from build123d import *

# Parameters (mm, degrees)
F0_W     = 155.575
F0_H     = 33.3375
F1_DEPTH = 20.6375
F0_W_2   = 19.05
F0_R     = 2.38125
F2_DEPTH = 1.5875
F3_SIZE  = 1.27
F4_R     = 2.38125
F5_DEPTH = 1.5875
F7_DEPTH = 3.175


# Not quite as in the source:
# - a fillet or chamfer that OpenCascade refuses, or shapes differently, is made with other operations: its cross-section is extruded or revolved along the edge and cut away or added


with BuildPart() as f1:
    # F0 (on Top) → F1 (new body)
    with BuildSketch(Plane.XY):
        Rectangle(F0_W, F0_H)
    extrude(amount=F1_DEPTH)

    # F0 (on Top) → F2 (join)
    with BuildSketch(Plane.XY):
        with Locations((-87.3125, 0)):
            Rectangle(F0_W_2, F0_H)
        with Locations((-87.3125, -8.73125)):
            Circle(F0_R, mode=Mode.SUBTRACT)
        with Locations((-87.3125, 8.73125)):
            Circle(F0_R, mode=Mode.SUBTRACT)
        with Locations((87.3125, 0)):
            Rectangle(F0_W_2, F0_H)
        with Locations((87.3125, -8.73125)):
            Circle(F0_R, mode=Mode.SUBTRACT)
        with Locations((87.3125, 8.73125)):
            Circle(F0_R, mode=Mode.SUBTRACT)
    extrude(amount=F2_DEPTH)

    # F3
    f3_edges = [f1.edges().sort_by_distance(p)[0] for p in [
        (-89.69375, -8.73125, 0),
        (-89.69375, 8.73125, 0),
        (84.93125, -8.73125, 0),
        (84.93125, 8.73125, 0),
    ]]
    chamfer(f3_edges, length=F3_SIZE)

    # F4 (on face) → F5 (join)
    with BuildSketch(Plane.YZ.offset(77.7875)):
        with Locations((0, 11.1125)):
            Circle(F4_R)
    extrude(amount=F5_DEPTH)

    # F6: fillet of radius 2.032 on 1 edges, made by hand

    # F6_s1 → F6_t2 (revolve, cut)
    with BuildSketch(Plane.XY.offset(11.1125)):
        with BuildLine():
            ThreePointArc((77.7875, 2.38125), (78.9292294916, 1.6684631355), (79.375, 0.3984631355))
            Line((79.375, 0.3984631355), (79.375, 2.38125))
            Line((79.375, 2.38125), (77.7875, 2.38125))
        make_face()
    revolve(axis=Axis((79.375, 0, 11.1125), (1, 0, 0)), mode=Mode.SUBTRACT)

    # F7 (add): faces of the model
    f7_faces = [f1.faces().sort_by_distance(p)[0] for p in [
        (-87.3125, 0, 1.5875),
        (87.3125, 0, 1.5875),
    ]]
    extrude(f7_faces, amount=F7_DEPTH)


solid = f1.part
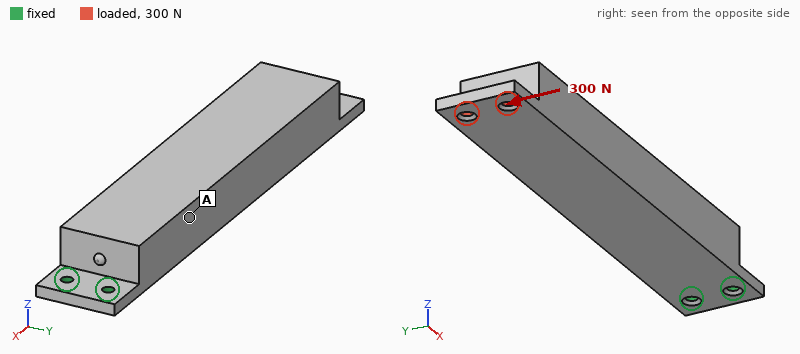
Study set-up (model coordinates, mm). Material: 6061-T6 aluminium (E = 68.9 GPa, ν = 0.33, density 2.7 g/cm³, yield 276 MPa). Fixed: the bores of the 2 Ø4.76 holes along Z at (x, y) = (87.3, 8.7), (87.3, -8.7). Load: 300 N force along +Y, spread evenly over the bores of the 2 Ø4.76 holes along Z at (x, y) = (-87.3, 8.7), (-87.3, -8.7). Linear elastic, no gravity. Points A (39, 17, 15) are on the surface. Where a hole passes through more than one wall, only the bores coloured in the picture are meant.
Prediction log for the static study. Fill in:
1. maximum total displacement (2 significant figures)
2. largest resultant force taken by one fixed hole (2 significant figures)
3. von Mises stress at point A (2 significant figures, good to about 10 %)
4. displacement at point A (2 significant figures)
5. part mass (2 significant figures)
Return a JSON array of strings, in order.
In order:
["0.30 mm", "2.6 kN", "9.6 MPa", "0.054 mm", "300 g"]
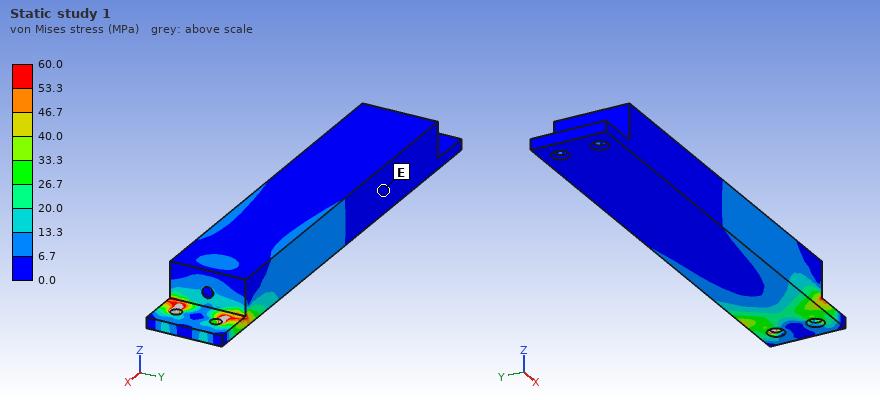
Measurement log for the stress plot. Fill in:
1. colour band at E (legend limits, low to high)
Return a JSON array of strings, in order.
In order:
["0.0 to 6.7 MPa"]
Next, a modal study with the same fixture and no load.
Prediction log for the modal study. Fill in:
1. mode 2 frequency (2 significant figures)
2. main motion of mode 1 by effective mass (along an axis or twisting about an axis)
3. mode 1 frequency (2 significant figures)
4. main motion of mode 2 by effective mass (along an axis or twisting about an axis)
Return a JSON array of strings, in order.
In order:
["570 Hz", "along Z", "120 Hz", "along Y"]
